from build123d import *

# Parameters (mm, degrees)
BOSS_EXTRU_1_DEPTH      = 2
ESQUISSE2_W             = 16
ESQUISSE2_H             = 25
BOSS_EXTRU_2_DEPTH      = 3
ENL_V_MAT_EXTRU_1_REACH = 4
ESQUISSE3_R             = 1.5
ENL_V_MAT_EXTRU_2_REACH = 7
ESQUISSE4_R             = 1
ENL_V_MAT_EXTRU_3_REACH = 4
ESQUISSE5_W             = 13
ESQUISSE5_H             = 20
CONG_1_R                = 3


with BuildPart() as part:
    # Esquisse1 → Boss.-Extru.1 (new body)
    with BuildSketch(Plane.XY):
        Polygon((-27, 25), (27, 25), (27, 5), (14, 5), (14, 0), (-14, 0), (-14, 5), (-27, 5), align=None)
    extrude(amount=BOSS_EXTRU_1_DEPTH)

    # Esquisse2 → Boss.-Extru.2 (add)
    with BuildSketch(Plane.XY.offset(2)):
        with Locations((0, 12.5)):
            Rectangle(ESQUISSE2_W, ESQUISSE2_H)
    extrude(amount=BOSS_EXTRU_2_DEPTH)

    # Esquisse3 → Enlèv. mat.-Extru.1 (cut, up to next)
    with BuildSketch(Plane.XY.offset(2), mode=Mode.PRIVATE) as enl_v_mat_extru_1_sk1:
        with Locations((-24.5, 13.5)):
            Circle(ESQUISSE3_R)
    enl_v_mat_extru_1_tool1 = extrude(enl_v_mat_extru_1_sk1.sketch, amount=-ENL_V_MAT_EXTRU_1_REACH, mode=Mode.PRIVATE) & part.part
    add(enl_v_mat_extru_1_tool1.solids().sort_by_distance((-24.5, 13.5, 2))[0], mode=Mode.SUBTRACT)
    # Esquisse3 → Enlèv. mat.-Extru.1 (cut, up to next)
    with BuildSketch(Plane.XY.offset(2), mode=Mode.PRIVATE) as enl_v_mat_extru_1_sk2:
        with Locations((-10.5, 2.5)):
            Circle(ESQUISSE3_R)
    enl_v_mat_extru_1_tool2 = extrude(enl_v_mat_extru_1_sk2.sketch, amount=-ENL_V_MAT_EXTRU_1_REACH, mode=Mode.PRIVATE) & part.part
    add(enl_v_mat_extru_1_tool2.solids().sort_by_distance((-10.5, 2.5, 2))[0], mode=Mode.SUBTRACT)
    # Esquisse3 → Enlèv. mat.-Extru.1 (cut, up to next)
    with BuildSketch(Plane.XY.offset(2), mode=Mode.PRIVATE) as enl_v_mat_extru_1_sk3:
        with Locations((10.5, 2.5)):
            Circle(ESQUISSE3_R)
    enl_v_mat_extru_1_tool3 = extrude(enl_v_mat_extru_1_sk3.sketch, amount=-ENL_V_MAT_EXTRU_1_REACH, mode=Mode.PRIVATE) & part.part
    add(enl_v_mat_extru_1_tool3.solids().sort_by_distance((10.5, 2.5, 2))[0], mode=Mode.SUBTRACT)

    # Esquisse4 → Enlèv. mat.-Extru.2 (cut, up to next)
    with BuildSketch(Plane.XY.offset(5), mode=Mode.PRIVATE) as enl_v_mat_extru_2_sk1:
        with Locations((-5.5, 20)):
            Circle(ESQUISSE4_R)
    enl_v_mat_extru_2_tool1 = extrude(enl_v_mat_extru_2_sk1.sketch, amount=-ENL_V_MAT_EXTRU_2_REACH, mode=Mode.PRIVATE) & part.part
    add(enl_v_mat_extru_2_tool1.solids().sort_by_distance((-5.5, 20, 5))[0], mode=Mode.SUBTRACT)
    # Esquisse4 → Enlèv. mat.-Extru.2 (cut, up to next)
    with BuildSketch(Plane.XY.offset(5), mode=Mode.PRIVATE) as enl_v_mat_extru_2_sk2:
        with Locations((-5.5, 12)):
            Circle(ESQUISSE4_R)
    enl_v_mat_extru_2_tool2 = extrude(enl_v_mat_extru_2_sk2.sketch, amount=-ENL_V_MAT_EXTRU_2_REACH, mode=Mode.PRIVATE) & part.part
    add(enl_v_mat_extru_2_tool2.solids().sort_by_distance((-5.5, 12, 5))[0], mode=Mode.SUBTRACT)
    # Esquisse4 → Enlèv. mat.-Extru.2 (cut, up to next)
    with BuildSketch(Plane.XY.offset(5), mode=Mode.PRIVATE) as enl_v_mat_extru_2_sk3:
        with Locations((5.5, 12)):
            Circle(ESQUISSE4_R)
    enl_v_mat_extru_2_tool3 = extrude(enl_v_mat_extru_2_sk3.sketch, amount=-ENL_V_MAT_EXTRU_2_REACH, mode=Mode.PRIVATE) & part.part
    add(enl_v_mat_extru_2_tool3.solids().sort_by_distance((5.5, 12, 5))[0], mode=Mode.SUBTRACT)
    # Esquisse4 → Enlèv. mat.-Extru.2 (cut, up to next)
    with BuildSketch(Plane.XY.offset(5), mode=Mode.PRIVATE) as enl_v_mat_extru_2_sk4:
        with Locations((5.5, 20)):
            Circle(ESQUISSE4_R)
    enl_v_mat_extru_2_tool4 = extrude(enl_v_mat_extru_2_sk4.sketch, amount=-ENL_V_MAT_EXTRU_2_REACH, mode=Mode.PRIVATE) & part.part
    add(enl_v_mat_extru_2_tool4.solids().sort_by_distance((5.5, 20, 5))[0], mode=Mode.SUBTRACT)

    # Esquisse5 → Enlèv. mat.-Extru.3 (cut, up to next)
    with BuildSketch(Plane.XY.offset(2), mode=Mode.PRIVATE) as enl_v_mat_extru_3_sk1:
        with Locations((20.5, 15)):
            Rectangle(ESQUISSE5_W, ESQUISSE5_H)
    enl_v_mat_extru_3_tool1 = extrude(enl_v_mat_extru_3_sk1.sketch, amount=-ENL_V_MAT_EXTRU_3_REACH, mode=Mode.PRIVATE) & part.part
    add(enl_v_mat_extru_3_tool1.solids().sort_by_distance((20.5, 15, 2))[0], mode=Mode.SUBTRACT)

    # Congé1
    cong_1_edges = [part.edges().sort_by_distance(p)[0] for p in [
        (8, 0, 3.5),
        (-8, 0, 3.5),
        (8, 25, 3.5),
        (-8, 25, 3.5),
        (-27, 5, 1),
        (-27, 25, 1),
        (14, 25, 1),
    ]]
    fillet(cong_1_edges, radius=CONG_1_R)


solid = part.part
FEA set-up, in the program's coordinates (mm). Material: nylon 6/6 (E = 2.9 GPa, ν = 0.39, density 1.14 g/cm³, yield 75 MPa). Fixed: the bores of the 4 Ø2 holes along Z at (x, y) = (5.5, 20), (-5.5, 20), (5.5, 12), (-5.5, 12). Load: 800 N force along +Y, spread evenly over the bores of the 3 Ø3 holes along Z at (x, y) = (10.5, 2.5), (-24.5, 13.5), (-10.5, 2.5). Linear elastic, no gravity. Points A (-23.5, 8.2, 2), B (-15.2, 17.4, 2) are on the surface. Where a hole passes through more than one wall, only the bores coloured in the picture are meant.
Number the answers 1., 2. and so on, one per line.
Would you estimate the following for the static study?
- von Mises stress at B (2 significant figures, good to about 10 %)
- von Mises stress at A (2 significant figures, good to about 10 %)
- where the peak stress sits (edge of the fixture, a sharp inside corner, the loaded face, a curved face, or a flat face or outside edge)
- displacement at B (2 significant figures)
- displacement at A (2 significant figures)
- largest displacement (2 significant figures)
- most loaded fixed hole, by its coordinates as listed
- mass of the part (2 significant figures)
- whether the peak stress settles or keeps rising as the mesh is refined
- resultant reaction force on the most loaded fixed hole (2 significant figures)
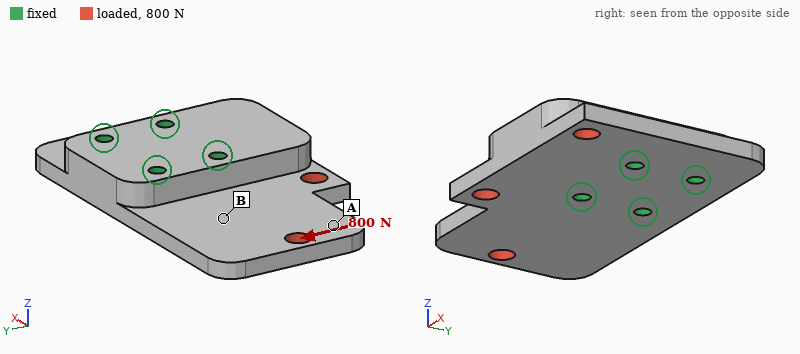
1. 18 MPa
2. 9.4 MPa
3. edge of the fixture
4. 0.16 mm
5. 0.35 mm
6. 0.43 mm
7. (-5.5, 12)
8. 3.4 g
9. keeps rising
10. 510 N
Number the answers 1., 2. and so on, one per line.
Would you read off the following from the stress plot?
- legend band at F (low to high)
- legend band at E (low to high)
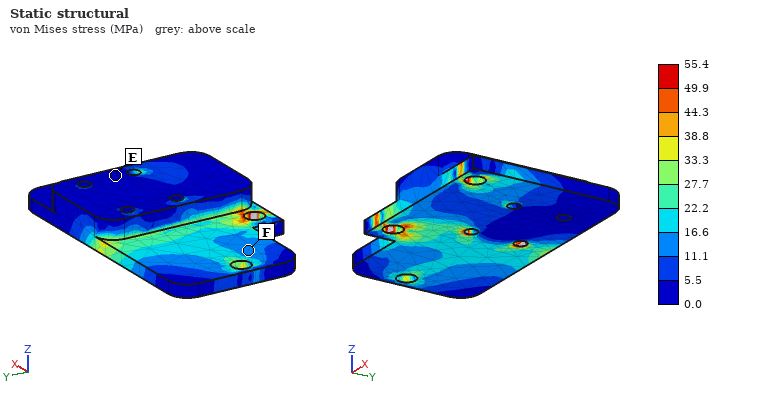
1. 11.1 to 16.6 MPa
2. 0.0 to 5.5 MPa
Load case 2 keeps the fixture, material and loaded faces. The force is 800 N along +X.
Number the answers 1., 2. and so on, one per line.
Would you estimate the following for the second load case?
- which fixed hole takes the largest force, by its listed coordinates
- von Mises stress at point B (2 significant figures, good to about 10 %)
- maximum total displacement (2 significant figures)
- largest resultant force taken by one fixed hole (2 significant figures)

1. (-5.5, 12)
2. 10.0 MPa
3. 0.23 mm
4. 570 N
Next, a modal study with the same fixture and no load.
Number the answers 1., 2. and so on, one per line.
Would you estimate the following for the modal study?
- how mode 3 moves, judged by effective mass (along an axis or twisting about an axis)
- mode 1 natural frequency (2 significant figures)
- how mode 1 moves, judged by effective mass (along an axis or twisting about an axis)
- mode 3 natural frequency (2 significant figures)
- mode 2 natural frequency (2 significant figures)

1. along Z
2. 1400 Hz
3. along Z
4. 7100 Hz
5. 3200 Hz
